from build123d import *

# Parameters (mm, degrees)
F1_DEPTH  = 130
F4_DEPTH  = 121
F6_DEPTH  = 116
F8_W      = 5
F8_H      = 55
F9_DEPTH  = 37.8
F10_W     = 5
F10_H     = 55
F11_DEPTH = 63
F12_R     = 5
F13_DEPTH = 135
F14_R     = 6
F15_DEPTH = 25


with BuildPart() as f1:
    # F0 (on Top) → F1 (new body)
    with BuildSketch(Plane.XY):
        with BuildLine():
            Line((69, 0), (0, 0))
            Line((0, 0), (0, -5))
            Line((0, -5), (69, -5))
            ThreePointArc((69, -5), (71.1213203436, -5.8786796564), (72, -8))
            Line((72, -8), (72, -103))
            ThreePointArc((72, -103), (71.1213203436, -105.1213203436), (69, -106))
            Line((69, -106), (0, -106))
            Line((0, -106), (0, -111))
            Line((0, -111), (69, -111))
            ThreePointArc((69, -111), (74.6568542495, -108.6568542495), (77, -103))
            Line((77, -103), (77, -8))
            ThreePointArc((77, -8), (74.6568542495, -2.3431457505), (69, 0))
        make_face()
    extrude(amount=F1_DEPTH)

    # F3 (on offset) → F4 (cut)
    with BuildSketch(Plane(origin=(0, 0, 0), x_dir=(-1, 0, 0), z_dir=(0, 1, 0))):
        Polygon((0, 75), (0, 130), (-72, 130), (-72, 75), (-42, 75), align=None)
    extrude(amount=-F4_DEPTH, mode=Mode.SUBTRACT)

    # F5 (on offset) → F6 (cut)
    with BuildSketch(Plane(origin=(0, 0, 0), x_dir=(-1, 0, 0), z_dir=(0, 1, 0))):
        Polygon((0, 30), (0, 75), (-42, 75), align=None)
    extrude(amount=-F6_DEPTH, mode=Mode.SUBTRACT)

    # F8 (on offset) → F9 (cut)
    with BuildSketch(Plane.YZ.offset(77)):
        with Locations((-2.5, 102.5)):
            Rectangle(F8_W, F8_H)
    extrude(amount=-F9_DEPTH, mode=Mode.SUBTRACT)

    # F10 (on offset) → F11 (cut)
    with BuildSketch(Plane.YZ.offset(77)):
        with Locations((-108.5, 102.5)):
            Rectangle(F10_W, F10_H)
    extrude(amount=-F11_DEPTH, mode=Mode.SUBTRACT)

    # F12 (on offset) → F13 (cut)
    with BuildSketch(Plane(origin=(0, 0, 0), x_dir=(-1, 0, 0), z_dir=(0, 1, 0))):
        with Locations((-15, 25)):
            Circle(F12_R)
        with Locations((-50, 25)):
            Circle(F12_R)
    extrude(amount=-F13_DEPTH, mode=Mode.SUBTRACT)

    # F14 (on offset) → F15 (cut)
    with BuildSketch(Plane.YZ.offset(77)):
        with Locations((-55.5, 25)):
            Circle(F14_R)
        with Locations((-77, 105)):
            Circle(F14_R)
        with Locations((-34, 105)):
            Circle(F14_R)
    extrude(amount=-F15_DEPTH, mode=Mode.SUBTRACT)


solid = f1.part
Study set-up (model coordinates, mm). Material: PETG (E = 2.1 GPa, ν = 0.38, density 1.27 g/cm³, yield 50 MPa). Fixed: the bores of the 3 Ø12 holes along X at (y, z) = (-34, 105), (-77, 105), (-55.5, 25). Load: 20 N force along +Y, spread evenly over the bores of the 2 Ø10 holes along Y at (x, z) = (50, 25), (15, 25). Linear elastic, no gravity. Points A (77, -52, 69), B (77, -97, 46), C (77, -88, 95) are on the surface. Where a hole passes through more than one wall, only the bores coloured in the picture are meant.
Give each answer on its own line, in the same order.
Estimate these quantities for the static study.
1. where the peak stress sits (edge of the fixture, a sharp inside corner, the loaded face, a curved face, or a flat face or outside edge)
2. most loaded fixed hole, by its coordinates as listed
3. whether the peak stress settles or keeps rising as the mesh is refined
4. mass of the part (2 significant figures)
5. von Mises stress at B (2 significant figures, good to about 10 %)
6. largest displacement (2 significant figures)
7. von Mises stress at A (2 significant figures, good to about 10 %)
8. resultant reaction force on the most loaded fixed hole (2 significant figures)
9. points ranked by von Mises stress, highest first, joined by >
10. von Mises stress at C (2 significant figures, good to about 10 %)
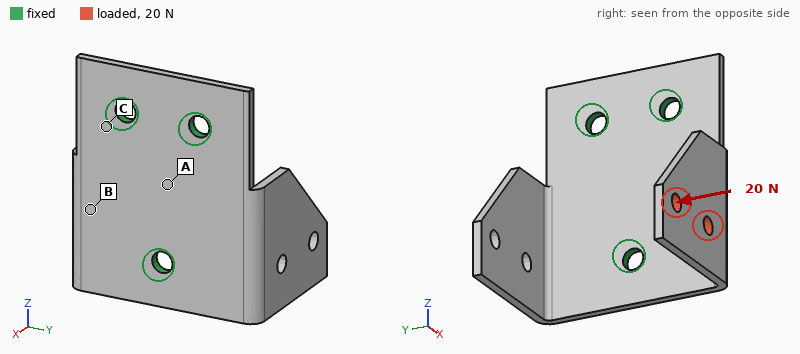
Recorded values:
a sharp inside corner
(-55.5, 25)
keeps rising
140 g
2.2 MPa
2.2 mm
0.36 MPa
19 N
B > C > A
1.4 MPa
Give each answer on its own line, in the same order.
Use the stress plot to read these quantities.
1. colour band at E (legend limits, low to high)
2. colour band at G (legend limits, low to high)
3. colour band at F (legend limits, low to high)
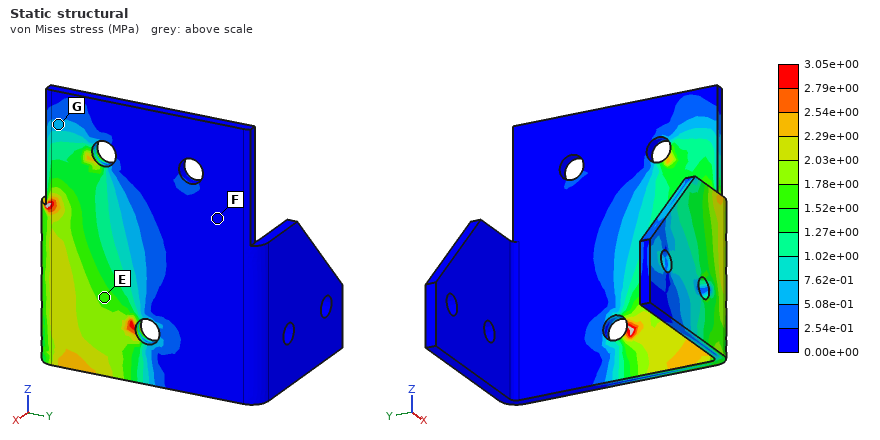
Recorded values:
1.52e+00 to 1.78e+00 MPa
5.08e-01 to 7.62e-01 MPa
0.00e+00 to 2.54e-01 MPa
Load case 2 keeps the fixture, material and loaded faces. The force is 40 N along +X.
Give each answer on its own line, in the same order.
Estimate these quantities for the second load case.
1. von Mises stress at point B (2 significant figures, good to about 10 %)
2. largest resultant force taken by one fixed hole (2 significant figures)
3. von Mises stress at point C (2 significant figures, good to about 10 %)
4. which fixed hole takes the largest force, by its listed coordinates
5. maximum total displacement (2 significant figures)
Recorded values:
2.0 MPa
35 N
2.1 MPa
(-55.5, 25)
2.1 mm
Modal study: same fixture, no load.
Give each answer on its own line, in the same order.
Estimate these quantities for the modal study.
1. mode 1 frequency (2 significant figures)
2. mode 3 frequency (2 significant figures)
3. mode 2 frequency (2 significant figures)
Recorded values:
120 Hz
250 Hz
130 Hz
